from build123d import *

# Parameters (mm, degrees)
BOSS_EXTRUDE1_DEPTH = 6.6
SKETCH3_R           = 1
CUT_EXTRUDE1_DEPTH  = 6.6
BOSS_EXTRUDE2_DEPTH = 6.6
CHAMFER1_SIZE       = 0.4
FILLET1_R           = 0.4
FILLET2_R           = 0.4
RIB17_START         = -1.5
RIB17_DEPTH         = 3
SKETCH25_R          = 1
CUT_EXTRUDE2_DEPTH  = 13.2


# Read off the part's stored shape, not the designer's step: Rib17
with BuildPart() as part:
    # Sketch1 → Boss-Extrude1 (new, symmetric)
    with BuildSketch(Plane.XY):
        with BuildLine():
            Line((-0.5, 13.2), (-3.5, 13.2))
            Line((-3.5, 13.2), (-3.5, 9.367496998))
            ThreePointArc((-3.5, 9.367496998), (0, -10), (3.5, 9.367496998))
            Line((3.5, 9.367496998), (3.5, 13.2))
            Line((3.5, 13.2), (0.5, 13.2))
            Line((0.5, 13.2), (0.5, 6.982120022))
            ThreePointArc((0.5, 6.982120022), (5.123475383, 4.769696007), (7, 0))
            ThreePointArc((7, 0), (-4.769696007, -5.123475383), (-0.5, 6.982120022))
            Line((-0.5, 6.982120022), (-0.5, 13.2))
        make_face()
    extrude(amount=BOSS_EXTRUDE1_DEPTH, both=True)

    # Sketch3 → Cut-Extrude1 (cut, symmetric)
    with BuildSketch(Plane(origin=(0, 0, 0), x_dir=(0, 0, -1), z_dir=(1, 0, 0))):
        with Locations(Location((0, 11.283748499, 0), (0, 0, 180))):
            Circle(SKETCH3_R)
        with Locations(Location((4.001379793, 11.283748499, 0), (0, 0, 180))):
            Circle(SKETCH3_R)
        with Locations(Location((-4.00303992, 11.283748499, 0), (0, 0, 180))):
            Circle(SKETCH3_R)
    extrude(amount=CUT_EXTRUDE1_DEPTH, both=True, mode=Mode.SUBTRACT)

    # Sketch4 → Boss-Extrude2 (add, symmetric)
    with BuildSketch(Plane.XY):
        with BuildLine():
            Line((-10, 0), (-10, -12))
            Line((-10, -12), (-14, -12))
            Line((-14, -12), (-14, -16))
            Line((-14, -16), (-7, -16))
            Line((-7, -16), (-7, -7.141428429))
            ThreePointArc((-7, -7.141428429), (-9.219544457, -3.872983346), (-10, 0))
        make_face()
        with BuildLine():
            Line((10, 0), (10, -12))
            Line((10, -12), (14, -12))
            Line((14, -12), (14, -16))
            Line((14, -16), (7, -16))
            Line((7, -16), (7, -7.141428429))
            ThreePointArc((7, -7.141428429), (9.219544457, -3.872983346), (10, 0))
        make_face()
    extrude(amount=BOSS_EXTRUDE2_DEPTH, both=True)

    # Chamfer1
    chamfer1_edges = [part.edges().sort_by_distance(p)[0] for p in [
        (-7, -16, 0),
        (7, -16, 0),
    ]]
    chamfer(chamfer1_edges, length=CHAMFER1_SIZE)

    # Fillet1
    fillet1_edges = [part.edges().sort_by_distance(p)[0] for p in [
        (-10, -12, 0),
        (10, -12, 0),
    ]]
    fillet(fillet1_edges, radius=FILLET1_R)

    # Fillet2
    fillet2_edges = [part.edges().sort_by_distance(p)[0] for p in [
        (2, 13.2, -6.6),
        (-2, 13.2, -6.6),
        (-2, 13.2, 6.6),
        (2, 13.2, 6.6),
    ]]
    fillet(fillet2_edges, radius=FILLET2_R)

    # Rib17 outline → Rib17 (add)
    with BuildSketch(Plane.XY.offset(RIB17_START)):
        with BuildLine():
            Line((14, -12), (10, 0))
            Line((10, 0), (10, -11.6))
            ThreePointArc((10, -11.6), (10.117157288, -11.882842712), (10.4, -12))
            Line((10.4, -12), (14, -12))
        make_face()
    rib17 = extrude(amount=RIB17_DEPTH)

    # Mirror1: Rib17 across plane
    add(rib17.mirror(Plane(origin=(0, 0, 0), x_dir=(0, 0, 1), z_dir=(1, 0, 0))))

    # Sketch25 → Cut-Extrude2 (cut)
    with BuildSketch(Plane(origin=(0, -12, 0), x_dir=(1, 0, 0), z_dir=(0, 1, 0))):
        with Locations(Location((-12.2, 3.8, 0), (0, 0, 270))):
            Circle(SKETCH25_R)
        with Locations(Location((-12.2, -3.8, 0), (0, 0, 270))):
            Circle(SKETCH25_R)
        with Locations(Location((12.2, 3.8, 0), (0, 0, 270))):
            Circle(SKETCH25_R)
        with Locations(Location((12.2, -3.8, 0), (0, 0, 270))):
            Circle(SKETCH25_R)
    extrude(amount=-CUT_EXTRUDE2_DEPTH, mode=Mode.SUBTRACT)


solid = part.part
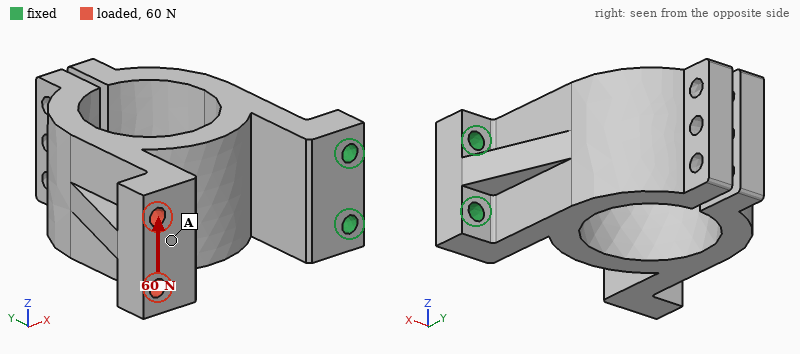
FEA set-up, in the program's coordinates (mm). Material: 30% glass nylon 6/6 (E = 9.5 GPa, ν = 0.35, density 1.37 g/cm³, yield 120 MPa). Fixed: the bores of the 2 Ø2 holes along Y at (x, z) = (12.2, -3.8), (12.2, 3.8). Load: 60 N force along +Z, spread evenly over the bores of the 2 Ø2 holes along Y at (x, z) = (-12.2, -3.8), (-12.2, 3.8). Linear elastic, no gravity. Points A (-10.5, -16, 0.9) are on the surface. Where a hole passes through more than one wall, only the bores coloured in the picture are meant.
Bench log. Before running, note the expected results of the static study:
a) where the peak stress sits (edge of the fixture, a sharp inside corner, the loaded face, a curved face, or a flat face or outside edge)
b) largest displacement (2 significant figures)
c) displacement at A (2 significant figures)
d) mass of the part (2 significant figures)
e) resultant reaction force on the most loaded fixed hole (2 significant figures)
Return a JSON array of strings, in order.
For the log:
["a curved face", "0.41 mm", "0.34 mm", "5.0 g", "160 N"]
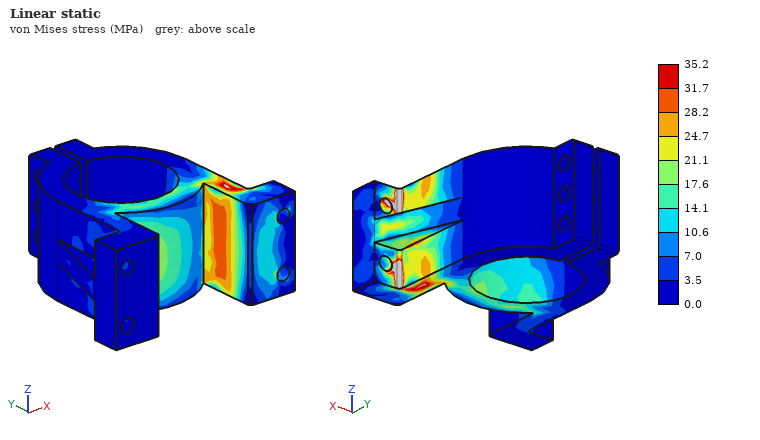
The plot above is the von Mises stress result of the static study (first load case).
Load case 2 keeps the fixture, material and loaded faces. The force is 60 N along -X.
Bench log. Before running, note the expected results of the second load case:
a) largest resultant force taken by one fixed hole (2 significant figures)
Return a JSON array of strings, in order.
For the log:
["30 N"]
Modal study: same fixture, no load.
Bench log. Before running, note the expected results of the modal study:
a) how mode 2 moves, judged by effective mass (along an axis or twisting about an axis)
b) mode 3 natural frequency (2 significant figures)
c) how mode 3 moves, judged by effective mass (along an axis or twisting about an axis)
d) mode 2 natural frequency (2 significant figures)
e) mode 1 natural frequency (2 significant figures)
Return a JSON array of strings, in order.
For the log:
["along Z", "2200 Hz", "along Z", "1600 Hz", "850 Hz"]
